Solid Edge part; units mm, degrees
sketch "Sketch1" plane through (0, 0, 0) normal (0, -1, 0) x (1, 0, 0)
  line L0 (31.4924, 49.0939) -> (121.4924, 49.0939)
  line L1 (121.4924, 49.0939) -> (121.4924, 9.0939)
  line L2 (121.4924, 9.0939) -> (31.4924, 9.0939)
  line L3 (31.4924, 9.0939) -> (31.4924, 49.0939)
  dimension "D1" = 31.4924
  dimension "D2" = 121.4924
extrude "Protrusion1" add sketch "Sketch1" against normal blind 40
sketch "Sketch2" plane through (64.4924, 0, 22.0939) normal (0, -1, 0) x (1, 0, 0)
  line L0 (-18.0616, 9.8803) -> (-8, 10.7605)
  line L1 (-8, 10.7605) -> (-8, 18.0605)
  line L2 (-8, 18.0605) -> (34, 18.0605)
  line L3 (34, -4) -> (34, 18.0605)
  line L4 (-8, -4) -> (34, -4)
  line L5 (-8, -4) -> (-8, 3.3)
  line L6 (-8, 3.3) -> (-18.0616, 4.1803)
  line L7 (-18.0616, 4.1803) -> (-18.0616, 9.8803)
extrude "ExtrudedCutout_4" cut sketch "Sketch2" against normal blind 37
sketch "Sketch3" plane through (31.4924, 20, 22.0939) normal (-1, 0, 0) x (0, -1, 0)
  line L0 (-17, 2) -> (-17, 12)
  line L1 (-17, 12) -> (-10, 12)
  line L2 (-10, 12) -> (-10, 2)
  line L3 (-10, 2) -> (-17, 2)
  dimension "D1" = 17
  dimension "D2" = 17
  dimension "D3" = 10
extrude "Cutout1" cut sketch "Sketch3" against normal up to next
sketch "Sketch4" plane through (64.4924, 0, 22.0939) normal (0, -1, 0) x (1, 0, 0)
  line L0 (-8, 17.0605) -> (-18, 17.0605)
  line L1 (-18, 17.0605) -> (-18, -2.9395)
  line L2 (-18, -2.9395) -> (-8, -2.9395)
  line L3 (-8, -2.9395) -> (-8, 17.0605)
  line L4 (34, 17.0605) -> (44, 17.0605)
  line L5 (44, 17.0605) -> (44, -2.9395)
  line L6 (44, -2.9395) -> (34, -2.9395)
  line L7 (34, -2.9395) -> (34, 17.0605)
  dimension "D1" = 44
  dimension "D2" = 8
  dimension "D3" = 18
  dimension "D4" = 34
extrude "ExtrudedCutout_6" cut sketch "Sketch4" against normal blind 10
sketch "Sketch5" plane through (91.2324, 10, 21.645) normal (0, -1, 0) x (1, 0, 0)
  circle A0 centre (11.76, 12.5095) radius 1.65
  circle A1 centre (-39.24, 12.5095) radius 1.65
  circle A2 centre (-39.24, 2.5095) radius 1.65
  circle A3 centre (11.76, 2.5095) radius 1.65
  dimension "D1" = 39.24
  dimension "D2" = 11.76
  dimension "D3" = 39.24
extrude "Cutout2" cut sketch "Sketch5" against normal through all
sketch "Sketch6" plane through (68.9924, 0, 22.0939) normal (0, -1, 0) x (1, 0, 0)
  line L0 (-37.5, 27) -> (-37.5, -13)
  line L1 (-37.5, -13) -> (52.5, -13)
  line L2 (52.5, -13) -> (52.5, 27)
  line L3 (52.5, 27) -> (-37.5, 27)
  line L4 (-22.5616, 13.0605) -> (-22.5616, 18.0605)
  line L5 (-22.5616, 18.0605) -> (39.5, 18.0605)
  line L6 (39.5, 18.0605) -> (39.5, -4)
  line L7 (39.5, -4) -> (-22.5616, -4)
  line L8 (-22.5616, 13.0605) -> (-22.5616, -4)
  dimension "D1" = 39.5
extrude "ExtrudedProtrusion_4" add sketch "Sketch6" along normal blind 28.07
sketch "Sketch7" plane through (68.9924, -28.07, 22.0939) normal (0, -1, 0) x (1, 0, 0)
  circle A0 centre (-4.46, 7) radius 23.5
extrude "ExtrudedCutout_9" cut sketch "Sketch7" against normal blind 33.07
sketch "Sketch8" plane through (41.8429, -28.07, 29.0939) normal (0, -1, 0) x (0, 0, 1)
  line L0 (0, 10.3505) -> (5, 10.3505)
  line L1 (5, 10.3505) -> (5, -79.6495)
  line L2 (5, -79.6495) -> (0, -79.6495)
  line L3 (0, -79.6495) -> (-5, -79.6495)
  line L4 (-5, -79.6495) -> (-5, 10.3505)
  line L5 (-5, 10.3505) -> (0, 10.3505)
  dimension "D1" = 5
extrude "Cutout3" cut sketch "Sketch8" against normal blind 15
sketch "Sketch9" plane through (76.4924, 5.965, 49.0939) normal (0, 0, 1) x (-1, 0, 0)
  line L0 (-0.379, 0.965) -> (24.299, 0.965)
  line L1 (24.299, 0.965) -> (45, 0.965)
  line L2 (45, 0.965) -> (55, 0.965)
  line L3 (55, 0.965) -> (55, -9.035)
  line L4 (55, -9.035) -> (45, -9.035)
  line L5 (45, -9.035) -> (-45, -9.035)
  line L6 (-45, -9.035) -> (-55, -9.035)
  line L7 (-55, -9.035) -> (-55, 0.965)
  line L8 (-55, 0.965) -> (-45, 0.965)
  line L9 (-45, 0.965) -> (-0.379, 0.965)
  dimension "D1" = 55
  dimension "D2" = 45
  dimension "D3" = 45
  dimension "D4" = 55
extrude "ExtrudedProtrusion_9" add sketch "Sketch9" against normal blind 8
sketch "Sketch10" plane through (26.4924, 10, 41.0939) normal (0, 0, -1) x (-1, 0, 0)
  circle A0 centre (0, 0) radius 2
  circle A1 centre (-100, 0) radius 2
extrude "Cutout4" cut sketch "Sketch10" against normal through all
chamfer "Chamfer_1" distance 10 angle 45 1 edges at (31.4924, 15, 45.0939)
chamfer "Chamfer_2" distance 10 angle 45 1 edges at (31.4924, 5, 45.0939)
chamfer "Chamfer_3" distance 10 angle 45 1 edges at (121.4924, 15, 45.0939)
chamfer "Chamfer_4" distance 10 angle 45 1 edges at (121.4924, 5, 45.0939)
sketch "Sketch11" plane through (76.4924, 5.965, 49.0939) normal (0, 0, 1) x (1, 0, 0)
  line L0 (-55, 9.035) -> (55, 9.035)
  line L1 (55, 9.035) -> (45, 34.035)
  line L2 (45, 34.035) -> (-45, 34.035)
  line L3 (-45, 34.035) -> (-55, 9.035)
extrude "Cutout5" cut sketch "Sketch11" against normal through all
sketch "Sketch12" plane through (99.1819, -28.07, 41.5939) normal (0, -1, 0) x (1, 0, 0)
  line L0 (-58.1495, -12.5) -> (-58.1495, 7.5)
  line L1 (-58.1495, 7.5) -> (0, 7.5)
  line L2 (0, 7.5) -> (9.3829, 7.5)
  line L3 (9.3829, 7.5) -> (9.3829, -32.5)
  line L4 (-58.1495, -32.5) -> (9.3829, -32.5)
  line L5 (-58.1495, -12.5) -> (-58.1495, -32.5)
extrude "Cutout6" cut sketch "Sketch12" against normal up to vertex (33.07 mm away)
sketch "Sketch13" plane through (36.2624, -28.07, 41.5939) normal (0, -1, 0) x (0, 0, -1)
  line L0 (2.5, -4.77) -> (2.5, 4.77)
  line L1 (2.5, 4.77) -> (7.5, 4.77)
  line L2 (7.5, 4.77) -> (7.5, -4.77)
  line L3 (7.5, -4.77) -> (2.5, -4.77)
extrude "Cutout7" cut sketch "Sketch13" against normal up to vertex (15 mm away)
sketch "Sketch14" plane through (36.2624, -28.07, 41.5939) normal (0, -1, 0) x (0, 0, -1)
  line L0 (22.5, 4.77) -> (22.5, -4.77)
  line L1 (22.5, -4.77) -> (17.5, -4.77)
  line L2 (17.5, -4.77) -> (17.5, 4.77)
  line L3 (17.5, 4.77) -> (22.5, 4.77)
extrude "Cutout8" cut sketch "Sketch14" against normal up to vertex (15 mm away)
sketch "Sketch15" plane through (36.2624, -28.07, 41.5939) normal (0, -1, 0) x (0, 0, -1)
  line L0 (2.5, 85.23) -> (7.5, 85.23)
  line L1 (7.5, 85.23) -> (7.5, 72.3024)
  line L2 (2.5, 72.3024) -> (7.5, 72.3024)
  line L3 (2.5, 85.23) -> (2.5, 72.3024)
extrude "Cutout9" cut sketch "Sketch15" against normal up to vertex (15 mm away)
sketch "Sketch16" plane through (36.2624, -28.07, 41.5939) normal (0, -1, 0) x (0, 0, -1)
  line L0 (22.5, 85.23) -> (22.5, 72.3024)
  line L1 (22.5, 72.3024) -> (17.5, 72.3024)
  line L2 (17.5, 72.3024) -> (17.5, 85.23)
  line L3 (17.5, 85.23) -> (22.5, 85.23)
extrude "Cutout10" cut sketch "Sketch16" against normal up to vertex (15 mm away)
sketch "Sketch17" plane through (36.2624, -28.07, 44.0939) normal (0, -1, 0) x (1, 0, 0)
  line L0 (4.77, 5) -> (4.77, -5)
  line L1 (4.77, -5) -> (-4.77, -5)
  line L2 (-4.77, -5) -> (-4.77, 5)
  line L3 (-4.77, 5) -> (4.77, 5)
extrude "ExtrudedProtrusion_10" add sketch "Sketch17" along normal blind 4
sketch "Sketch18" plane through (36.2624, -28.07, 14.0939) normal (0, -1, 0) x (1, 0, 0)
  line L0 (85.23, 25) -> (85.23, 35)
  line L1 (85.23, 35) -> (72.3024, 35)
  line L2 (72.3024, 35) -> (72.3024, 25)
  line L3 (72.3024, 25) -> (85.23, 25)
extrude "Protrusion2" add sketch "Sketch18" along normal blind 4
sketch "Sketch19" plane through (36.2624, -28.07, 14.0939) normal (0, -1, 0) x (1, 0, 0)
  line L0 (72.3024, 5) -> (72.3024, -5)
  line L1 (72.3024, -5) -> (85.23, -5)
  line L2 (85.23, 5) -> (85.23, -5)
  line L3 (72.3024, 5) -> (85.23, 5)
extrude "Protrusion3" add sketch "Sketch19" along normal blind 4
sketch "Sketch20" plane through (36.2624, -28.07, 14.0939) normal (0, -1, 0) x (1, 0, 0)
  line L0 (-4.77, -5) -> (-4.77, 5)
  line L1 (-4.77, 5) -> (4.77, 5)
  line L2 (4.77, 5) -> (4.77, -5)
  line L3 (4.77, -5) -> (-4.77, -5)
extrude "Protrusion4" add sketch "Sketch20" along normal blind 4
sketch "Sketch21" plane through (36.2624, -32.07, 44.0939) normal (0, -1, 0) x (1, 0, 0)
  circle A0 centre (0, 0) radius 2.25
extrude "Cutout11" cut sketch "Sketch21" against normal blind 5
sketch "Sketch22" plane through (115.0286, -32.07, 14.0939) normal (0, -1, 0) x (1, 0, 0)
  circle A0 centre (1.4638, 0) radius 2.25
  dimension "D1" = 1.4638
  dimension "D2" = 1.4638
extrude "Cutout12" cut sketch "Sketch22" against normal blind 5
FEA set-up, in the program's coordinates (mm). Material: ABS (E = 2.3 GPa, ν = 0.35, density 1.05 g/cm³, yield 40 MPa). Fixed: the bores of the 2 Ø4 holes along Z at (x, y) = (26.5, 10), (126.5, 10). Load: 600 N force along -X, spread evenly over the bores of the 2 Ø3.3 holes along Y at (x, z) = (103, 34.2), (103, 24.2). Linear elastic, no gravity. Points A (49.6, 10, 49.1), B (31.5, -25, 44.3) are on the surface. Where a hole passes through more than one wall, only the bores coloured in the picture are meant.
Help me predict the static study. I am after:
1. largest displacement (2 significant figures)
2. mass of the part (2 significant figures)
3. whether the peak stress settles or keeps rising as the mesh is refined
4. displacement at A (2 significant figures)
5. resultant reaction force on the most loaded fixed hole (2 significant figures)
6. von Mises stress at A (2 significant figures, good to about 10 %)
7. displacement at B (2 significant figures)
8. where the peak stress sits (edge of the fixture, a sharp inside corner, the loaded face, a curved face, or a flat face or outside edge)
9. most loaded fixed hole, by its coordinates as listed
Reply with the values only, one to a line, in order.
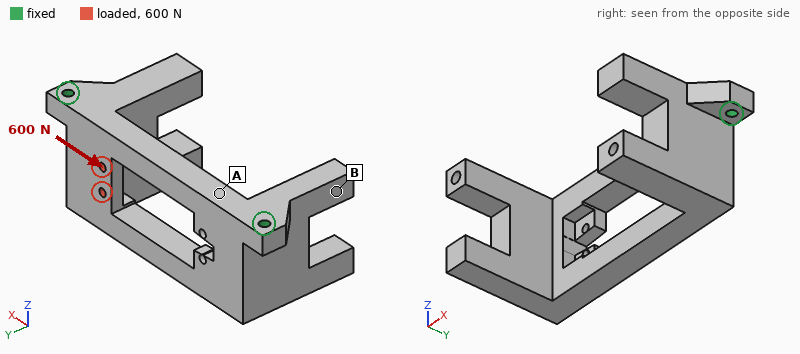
0.27 mm
54 g
keeps rising
0.068 mm
420 N
5.0 MPa
0.055 mm
edge of the fixture
(126.5, 10)
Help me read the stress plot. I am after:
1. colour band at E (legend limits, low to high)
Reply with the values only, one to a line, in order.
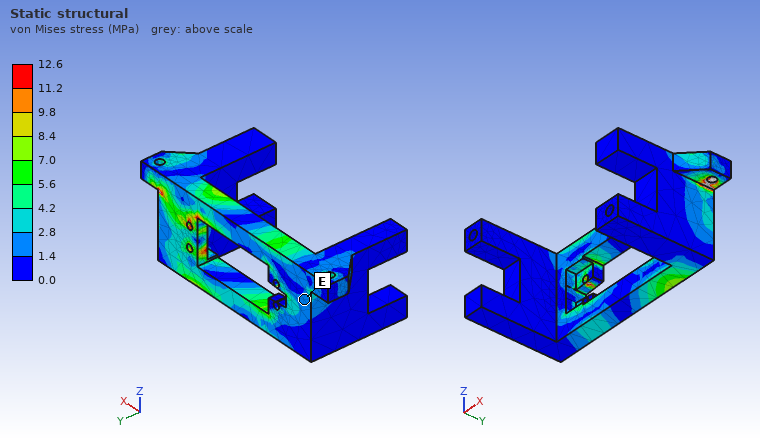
1.4 to 2.8 MPa
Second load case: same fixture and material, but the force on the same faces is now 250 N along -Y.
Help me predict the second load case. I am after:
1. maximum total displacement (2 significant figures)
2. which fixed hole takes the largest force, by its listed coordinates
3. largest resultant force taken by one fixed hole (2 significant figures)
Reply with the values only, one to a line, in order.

0.95 mm
(126.5, 10)
200 N
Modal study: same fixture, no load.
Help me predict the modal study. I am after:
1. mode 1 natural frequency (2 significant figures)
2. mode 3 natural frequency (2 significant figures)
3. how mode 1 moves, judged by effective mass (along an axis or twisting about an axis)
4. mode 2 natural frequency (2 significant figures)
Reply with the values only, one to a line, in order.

510 Hz
820 Hz
along Y
700 Hz
